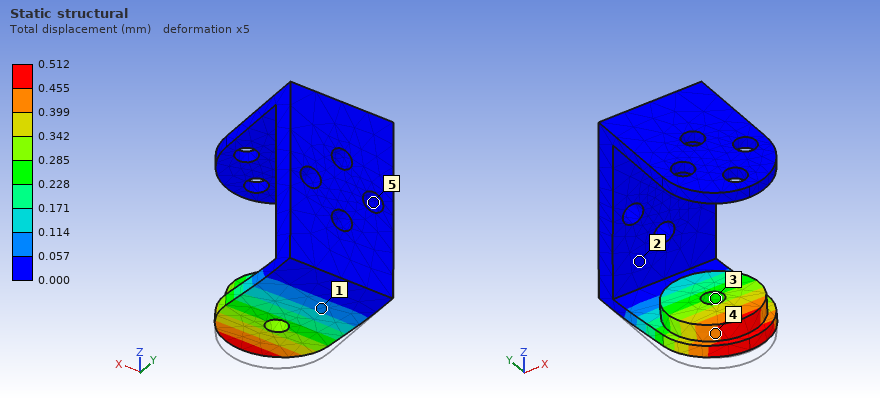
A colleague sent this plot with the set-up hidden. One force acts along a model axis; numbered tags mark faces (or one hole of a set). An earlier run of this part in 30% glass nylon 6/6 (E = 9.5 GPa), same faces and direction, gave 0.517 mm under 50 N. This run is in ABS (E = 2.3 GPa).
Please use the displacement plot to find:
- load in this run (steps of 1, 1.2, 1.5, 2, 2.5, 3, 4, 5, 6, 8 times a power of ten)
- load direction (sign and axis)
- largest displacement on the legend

12 N
+Z
0.512 mm
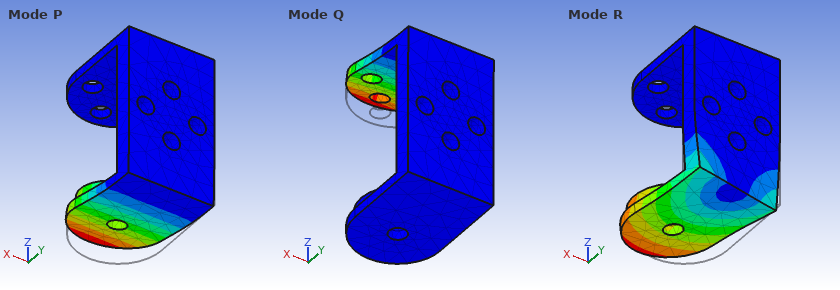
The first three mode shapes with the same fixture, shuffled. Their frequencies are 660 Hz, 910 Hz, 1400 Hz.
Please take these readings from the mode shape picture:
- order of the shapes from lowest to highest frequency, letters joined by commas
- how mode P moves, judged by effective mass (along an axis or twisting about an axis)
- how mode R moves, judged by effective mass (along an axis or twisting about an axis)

P, Q, R
along Z
along X
